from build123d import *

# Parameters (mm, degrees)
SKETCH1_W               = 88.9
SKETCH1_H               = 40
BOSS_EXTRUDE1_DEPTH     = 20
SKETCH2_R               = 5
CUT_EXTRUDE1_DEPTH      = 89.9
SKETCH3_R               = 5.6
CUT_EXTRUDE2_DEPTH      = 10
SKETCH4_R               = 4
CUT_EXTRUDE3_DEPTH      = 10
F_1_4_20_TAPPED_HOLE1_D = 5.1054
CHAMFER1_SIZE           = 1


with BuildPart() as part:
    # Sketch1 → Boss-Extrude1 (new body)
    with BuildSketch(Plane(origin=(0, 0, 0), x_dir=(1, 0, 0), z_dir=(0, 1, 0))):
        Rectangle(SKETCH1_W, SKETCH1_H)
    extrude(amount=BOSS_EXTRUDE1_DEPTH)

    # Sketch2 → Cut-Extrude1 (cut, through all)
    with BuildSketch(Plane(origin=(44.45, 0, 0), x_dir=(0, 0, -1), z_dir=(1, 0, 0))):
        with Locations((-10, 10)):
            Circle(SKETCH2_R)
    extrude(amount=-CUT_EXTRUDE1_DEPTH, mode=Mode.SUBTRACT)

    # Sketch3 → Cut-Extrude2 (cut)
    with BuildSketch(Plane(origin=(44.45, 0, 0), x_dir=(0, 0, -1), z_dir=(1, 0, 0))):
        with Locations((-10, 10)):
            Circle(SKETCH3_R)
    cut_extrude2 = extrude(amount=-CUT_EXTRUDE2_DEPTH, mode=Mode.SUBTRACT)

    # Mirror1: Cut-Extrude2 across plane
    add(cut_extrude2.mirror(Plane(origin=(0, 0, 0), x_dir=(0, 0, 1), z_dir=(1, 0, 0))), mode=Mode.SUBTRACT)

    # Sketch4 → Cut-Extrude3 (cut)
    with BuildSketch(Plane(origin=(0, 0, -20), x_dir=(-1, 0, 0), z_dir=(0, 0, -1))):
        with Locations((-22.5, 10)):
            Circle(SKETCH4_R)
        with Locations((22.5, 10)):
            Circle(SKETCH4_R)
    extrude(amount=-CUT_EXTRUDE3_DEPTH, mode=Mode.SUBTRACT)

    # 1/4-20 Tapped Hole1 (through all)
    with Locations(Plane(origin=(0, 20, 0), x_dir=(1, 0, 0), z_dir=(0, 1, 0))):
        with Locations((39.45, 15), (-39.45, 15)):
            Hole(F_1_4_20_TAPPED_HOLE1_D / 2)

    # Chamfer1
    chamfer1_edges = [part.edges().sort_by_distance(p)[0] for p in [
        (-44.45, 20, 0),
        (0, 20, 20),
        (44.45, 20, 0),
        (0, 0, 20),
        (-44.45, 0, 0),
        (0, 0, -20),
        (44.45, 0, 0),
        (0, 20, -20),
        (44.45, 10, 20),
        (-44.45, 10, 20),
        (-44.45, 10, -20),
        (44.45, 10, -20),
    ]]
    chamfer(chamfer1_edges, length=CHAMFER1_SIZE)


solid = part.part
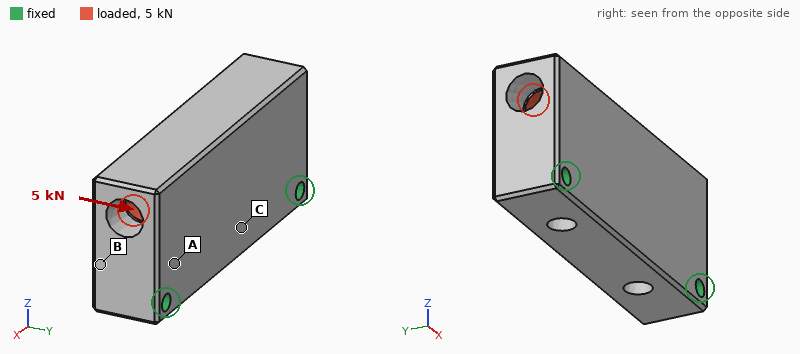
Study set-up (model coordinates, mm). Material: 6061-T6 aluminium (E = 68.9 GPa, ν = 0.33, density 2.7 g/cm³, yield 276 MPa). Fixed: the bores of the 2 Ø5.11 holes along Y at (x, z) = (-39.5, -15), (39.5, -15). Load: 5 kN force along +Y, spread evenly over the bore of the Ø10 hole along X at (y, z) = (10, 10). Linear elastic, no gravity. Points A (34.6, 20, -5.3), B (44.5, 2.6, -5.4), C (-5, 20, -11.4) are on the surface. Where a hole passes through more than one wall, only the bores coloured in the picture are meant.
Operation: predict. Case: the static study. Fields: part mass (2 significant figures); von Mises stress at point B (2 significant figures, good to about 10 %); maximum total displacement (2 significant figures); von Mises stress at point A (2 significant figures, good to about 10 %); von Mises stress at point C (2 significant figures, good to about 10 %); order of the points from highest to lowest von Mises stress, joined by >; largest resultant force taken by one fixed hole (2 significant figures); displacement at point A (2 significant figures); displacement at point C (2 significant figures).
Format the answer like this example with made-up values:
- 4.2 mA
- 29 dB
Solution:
- 170 g
- 20 MPa
- 56 µm
- 36 MPa
- 9.6 MPa
- A > B > C
- 2.5 kN
- 12 µm
- 16 µm
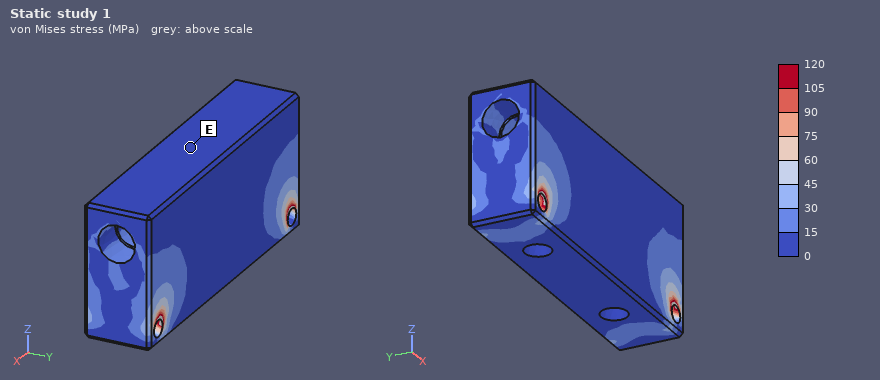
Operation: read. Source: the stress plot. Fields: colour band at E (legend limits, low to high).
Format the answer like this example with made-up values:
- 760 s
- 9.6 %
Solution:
- 0 to 15 MPa
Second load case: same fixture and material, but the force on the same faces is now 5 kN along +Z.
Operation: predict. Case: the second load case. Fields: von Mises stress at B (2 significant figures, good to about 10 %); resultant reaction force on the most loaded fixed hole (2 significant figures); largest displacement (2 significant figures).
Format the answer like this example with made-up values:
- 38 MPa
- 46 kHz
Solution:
- 3.5 MPa
- 2.9 kN
- 7.9 µm
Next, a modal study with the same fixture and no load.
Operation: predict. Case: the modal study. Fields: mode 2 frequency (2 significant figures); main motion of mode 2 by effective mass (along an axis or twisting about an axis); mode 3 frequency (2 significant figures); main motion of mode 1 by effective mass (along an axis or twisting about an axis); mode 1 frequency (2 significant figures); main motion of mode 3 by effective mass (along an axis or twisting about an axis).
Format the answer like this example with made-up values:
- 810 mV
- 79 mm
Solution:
- 12 kHz
- along Y
- 12 kHz
- along Y
- 6300 Hz
- twisting about Z
